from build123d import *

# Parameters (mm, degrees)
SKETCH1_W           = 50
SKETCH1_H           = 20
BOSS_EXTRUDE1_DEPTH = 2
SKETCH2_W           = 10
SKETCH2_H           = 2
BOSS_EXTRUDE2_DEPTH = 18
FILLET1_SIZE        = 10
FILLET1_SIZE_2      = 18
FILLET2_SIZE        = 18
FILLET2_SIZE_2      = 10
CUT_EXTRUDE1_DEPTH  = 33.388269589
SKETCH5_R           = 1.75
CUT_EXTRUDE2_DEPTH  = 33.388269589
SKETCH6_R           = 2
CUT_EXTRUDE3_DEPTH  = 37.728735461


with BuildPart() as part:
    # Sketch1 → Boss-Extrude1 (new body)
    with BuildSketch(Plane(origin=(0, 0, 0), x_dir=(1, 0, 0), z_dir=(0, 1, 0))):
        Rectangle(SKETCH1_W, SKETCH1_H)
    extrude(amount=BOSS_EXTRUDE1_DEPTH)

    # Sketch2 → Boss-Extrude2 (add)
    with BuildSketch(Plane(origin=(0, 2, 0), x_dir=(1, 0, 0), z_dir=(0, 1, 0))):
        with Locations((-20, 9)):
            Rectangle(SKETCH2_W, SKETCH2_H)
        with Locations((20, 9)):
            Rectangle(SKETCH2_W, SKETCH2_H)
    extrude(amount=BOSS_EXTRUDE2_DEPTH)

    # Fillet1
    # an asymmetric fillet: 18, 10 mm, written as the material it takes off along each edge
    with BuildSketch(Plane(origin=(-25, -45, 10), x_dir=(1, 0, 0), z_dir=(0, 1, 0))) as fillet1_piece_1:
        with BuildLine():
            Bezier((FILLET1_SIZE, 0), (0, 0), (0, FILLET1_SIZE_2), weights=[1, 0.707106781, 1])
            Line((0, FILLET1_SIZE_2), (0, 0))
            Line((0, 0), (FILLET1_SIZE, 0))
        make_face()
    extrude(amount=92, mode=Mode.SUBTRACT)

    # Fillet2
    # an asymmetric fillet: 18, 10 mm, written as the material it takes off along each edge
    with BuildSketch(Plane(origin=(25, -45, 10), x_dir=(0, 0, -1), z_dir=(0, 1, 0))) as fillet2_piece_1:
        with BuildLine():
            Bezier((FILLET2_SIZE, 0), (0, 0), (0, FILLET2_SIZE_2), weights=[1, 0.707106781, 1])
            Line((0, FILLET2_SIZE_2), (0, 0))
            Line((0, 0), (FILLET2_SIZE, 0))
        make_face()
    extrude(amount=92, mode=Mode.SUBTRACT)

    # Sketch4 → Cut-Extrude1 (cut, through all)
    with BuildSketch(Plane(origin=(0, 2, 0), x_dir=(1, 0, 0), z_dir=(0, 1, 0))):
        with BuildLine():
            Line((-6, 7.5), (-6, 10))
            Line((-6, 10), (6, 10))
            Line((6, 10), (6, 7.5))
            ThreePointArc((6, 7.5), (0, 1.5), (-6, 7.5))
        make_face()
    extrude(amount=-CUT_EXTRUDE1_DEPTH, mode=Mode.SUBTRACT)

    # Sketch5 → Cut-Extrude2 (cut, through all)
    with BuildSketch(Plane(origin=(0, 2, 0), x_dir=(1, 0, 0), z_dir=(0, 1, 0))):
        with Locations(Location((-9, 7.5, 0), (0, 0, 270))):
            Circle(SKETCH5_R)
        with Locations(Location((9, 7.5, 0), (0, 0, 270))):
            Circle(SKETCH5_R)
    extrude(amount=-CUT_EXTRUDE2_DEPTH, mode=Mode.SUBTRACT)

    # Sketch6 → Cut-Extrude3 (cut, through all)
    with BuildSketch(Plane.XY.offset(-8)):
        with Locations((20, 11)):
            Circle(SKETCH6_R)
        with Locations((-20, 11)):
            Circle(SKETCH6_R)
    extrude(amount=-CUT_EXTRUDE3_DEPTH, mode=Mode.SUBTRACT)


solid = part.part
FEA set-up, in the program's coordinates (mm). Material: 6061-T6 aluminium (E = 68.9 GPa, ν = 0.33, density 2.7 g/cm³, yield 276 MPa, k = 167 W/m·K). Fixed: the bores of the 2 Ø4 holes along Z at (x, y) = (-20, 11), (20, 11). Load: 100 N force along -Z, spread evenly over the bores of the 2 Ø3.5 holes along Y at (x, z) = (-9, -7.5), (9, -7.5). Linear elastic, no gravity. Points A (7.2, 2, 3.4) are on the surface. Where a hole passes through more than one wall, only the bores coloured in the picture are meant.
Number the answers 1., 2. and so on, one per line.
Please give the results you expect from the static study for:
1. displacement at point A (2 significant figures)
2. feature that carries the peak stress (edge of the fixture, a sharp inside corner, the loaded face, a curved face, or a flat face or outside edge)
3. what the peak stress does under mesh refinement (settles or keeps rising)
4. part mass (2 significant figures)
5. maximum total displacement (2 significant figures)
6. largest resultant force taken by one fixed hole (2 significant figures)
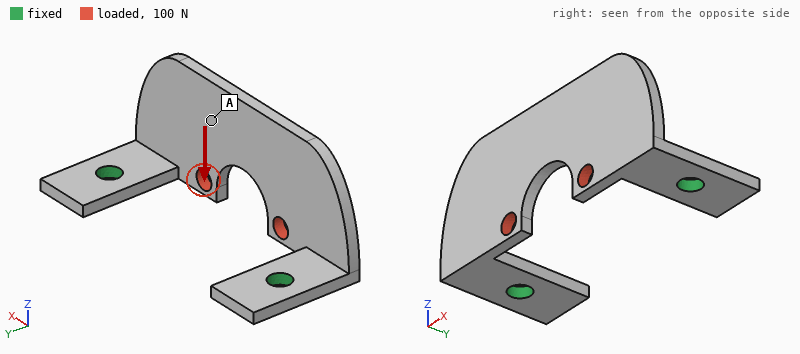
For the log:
1. 55 µm
2. edge of the fixture
3. keeps rising
4. 6.2 g
5. 83 µm
6. 54 N
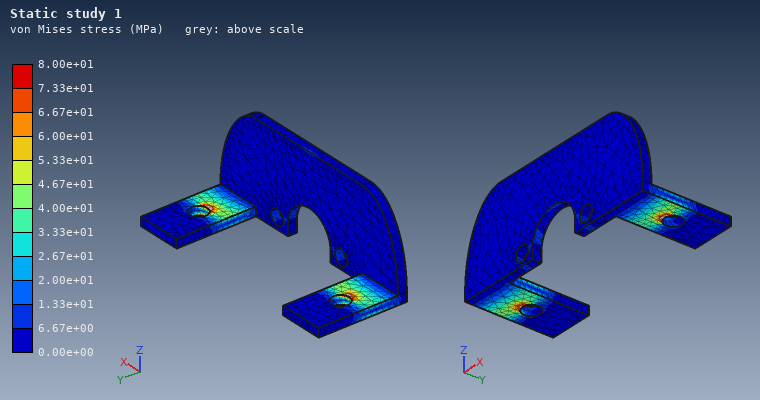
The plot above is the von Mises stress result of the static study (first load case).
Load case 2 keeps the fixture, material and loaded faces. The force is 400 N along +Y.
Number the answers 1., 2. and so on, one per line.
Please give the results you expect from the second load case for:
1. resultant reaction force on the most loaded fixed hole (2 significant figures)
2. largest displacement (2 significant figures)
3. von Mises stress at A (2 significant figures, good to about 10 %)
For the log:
1. 220 N
2. 0.17 mm
3. 41 MPa
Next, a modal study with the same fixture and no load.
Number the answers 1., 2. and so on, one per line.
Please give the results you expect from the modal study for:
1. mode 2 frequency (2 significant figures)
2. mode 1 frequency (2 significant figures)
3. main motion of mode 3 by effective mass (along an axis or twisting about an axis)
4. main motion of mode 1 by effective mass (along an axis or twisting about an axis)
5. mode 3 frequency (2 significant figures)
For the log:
1. 4300 Hz
2. 1900 Hz
3. along Z
4. along Y
5. 6600 Hz
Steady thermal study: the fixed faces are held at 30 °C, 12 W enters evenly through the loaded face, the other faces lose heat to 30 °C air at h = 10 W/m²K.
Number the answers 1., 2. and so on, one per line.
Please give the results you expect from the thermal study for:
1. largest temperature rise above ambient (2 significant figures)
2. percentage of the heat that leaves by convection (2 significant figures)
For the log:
1. 39 K
2. 4.0 %
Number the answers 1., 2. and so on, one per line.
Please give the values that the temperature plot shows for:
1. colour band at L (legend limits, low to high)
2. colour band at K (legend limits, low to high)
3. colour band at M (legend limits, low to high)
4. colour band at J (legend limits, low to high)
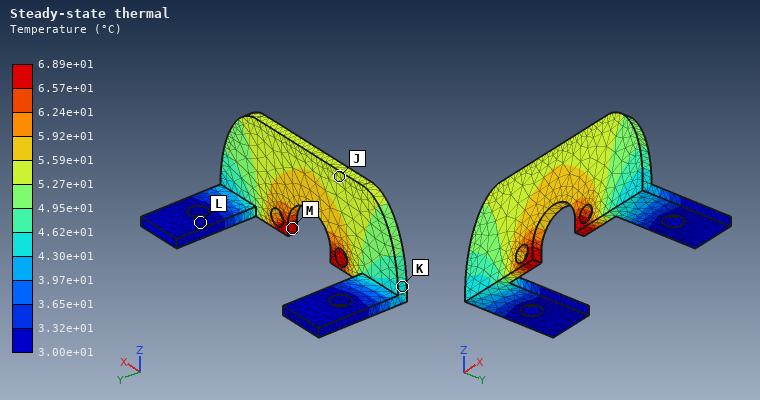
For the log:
1. 3.00e+01 to 3.32e+01 °C
2. 4.30e+01 to 4.62e+01 °C
3. 6.57e+01 to 6.89e+01 °C
4. 5.27e+01 to 5.59e+01 °C
